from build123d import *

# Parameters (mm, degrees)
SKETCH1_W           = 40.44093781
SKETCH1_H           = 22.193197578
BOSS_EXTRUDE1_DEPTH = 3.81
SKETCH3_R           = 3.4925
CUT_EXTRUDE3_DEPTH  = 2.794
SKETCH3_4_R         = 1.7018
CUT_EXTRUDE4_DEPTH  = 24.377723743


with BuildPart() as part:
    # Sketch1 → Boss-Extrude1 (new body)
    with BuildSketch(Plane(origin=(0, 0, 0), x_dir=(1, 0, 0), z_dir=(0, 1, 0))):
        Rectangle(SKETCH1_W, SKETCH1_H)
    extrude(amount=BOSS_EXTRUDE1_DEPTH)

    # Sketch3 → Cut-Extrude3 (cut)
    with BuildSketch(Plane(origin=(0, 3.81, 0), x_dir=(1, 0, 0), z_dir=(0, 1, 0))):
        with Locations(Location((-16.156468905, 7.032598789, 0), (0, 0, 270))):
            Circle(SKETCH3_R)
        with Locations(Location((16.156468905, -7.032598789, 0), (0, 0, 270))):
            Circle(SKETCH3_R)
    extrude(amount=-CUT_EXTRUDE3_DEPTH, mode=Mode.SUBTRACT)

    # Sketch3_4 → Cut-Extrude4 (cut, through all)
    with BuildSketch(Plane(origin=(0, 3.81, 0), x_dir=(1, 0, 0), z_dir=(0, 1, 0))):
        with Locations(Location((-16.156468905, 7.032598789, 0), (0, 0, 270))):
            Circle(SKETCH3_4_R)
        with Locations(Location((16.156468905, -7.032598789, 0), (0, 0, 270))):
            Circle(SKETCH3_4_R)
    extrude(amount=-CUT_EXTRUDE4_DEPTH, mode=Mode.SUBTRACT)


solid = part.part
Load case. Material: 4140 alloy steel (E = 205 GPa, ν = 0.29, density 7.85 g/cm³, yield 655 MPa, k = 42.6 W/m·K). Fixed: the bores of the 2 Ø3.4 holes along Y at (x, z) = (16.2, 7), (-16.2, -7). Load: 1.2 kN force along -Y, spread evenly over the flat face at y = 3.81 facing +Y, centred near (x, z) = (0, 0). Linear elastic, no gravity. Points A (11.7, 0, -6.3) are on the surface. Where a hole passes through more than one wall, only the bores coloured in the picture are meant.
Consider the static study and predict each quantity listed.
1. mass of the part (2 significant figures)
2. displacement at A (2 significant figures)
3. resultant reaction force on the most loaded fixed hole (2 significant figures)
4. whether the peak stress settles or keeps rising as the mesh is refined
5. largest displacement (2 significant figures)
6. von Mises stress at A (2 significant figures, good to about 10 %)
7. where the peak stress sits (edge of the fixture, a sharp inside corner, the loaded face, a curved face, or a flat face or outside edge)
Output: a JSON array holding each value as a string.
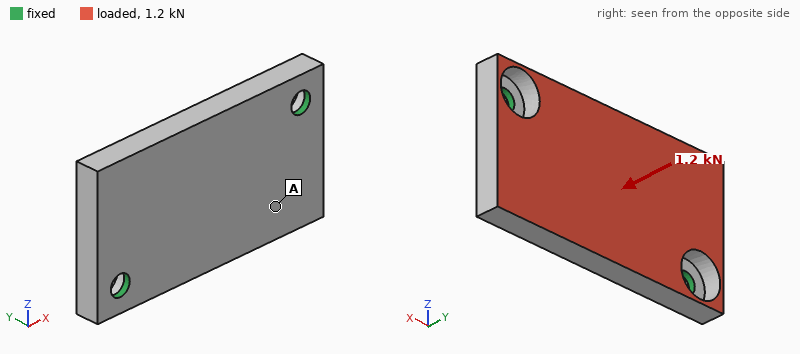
["25 g", "23 µm", "1.0 kN", "keeps rising", "29 µm", "35 MPa", "edge of the fixture"]
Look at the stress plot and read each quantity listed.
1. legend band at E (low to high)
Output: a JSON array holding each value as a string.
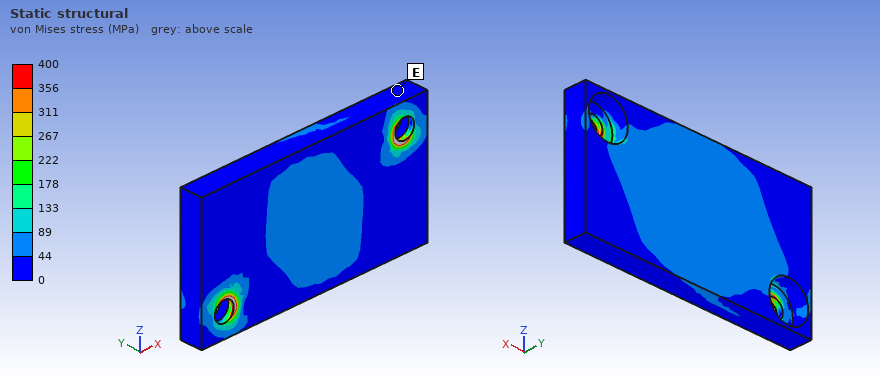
["0 to 44 MPa"]
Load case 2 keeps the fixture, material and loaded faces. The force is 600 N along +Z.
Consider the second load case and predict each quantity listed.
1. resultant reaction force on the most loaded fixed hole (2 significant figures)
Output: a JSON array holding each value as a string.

["300 N"]
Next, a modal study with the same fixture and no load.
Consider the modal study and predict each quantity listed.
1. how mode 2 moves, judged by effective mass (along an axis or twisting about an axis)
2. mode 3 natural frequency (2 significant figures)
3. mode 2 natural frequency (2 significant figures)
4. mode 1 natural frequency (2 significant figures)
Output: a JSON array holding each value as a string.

["along Y", "14 kHz", "7800 Hz", "4100 Hz"]
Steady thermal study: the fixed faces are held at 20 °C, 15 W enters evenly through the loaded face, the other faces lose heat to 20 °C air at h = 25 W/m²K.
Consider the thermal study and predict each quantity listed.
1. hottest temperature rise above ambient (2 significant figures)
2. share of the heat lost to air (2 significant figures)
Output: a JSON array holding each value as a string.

["49 K", "9.4 %"]
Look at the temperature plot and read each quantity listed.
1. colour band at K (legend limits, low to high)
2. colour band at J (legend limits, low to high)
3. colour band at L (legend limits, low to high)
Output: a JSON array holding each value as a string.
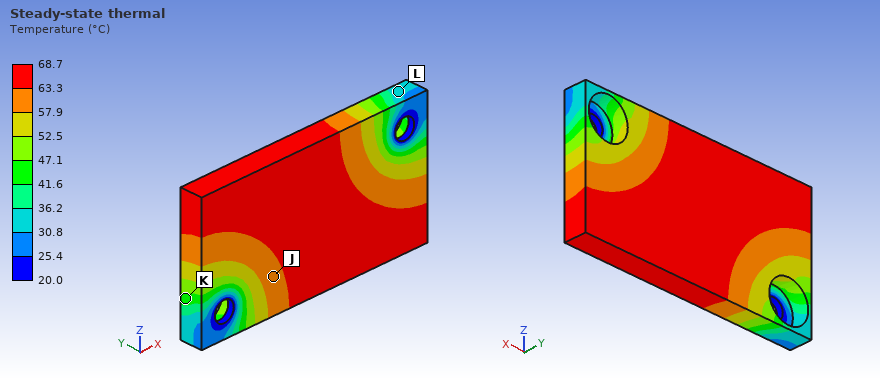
["41.6 to 47.1 °C", "57.9 to 63.3 °C", "30.8 to 36.2 °C"]
